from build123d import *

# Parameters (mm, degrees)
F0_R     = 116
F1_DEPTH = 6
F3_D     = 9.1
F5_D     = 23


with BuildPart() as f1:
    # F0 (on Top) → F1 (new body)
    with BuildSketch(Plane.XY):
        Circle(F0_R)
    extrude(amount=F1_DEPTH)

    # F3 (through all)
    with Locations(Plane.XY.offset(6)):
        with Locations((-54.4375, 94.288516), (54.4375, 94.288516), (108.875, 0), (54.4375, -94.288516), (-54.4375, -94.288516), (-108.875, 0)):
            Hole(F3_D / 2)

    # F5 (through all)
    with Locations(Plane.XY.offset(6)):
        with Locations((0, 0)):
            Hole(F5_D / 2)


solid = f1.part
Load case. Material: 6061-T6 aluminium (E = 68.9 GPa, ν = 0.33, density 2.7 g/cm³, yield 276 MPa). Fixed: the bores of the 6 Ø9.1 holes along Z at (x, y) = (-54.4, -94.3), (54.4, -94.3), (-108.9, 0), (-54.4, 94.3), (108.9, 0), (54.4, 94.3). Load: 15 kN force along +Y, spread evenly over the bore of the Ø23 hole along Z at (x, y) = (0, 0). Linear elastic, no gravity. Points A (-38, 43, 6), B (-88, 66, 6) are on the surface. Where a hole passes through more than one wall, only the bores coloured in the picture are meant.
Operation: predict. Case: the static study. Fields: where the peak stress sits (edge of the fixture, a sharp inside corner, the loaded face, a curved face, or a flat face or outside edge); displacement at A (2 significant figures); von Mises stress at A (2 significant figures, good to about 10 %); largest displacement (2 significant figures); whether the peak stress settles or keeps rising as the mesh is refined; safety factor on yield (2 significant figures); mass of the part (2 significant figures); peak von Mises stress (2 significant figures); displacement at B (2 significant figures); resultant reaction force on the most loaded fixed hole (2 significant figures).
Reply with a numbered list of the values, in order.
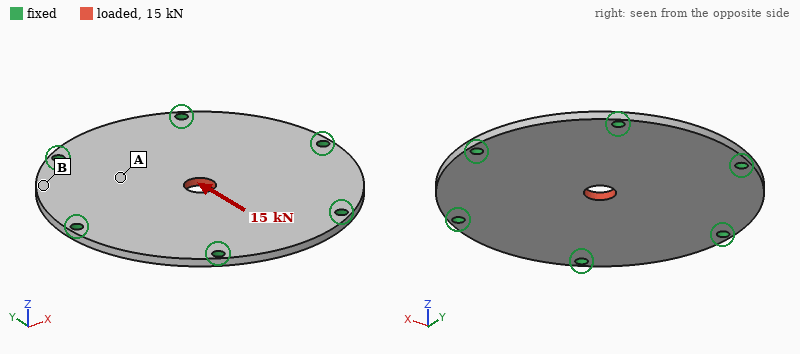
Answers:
1. the loaded face
2. 11 µm
3. 12 MPa
4. 28 µm
5. settles
6. 4.6
7. 670 g
8. 60 MPa
9. 6.3 µm
10. 3.3 kN
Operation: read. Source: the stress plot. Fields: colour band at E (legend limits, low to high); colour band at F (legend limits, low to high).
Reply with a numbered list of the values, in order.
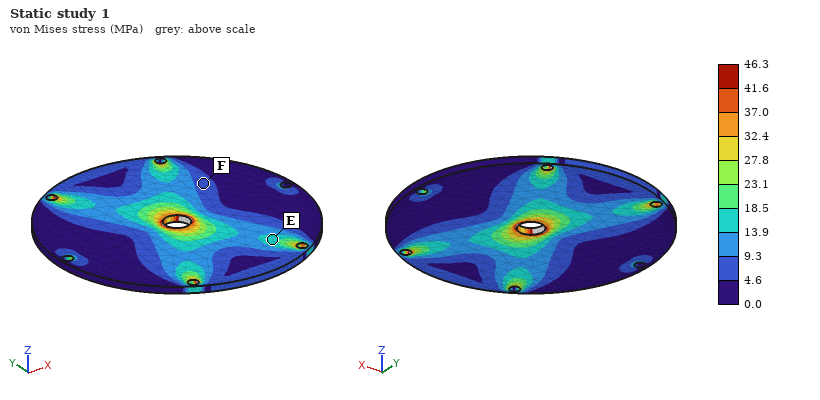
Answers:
1. 13.9 to 18.5 MPa
2. 4.6 to 9.3 MPa
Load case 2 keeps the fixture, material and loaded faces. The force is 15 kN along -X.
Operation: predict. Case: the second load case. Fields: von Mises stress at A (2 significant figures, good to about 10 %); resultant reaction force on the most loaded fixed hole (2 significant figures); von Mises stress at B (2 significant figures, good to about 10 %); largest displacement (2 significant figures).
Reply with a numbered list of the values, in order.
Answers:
1. 8.1 MPa
2. 3.7 kN
3. 5.9 MPa
4. 28 µm
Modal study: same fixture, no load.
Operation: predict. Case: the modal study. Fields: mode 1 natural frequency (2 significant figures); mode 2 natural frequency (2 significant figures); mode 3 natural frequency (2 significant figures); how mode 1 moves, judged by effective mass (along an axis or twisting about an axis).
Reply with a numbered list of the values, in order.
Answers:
1. 1000 Hz
2. 2100 Hz
3. 2100 Hz
4. along Z
